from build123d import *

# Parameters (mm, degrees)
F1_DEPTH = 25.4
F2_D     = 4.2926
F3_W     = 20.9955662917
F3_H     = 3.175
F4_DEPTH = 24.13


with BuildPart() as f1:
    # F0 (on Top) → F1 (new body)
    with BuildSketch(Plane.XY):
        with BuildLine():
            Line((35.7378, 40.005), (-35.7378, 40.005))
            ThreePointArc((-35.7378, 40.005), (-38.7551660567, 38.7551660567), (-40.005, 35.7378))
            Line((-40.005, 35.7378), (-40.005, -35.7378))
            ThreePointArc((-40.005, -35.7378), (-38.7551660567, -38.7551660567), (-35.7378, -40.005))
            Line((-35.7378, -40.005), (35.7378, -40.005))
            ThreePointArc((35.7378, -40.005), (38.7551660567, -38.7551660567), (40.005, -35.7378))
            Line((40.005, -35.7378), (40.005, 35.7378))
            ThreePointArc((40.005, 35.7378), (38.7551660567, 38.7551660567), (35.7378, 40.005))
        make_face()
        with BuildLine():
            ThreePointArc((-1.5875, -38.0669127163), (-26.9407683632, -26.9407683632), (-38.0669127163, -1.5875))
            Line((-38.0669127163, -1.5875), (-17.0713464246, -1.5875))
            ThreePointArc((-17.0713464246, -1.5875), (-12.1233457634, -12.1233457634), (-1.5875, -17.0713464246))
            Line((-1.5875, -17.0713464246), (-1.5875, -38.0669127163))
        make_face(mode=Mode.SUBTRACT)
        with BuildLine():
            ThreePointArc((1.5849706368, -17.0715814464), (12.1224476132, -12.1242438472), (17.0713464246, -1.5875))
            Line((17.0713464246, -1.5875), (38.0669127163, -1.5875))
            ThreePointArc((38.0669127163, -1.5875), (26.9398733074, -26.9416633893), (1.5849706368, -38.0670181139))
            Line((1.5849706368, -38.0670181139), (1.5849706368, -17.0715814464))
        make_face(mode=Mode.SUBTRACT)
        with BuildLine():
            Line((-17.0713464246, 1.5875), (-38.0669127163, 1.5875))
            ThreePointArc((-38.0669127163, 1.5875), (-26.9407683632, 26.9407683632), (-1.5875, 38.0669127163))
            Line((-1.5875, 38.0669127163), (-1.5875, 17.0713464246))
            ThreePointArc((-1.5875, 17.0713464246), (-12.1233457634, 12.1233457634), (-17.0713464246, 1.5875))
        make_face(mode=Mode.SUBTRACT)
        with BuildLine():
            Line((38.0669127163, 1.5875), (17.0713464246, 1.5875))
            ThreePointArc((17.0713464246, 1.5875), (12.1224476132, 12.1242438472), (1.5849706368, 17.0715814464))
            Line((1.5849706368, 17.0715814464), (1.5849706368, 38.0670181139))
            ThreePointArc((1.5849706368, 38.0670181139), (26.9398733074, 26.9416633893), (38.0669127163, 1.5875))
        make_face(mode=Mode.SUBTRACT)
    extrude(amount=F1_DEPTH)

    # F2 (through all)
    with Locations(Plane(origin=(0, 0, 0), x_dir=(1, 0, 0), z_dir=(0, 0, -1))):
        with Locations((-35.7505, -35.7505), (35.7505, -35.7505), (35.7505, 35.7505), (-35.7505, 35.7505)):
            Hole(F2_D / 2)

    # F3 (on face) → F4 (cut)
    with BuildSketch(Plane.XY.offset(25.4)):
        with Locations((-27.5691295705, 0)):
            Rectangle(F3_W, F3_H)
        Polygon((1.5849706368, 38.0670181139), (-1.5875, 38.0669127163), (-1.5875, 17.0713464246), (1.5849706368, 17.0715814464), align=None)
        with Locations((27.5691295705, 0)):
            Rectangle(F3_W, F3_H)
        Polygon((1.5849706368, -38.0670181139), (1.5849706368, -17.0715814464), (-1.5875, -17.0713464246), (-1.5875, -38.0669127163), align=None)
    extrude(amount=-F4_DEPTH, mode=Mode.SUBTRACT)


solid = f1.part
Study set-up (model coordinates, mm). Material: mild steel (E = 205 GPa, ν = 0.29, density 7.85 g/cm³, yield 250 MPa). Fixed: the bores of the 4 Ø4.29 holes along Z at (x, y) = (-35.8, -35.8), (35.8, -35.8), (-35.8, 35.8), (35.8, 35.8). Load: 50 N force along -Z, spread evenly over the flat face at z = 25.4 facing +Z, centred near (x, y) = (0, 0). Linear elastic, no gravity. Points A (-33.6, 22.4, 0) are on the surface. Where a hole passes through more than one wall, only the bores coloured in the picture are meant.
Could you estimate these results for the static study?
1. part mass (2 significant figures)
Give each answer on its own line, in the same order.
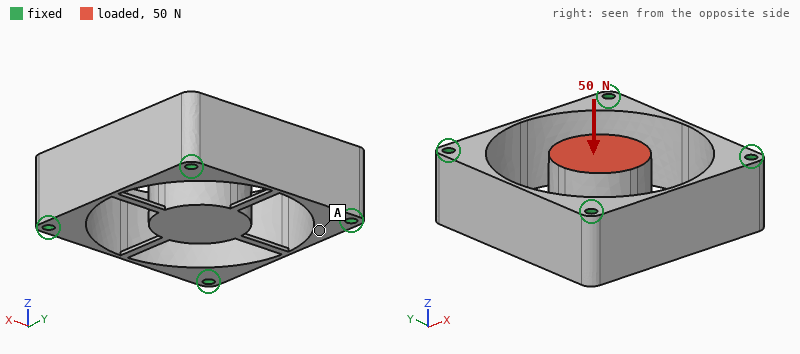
540 g
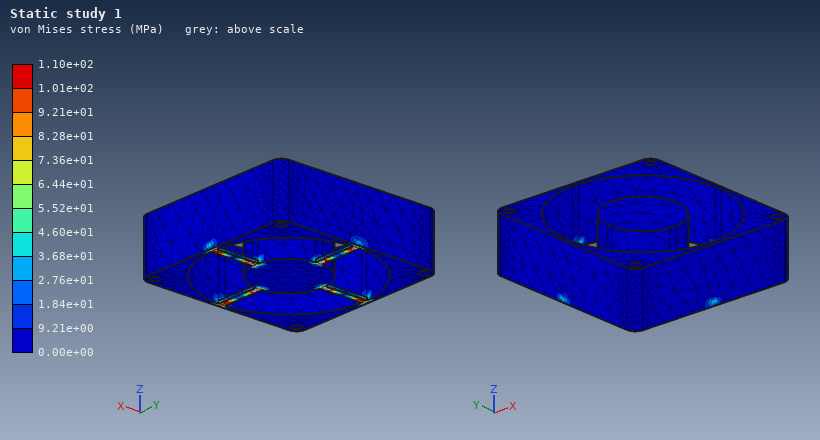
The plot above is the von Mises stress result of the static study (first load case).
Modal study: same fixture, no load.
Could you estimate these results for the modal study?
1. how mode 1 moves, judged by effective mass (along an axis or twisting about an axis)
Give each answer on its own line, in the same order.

along Z
